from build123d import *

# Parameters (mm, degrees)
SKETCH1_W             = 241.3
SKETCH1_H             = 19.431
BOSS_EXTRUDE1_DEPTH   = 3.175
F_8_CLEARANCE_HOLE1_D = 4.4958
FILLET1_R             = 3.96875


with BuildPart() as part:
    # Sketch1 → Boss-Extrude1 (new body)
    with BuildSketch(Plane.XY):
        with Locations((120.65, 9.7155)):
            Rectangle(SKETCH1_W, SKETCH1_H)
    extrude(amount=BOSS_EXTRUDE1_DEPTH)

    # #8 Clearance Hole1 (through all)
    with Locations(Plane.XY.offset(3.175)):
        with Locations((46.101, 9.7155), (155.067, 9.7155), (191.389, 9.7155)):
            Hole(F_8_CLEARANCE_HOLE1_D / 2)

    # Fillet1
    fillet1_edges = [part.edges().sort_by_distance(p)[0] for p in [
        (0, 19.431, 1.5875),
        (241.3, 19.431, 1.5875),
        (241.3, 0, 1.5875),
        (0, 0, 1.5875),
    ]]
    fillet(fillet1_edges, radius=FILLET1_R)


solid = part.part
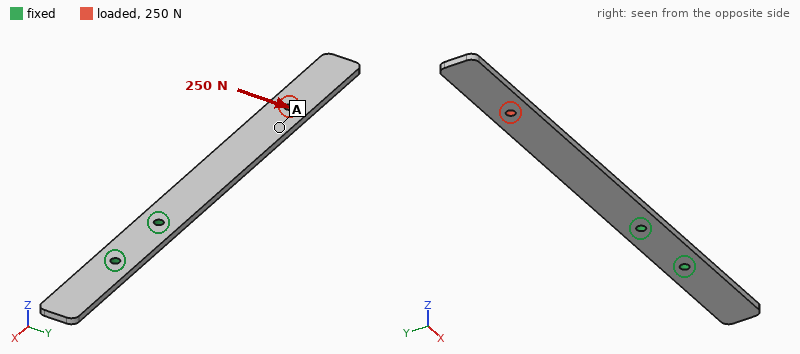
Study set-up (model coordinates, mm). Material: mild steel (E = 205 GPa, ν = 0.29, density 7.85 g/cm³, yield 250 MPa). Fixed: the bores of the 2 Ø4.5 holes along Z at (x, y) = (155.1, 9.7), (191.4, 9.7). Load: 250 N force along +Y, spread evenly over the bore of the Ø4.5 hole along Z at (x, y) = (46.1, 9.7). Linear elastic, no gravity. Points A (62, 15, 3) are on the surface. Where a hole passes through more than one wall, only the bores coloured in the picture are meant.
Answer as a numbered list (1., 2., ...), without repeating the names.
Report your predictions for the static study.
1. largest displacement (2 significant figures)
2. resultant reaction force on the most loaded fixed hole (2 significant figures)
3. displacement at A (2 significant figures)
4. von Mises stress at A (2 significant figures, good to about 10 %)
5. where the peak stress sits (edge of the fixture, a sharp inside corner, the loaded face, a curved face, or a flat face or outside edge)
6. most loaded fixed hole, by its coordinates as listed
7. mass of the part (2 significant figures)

1. 0.54 mm
2. 750 N
3. 0.27 mm
4. 13 MPa
5. edge of the fixture
6. (155.1, 9.7)
7. 120 g
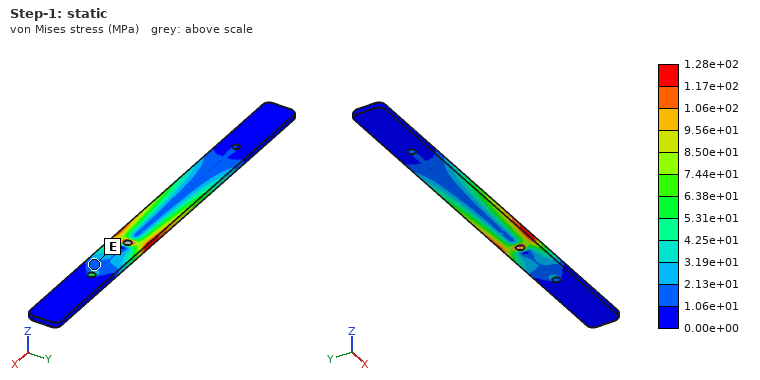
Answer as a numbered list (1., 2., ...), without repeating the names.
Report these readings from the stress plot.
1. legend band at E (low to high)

1. 1.06e+01 to 2.13e+01 MPa
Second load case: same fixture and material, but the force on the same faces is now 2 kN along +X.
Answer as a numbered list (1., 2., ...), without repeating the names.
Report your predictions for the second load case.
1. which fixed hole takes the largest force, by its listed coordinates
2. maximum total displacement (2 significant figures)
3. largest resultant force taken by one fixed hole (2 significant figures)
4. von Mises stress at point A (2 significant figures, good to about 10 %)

1. (155.1, 9.7)
2. 19 µm
3. 1.8 kN
4. 33 MPa
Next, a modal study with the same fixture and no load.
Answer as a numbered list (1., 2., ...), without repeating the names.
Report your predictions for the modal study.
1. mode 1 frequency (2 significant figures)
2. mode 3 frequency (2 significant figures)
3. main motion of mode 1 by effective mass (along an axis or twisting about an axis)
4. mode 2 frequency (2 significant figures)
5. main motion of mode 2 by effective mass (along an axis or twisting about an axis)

1. 110 Hz
2. 690 Hz
3. along Z
4. 600 Hz
5. along Y
